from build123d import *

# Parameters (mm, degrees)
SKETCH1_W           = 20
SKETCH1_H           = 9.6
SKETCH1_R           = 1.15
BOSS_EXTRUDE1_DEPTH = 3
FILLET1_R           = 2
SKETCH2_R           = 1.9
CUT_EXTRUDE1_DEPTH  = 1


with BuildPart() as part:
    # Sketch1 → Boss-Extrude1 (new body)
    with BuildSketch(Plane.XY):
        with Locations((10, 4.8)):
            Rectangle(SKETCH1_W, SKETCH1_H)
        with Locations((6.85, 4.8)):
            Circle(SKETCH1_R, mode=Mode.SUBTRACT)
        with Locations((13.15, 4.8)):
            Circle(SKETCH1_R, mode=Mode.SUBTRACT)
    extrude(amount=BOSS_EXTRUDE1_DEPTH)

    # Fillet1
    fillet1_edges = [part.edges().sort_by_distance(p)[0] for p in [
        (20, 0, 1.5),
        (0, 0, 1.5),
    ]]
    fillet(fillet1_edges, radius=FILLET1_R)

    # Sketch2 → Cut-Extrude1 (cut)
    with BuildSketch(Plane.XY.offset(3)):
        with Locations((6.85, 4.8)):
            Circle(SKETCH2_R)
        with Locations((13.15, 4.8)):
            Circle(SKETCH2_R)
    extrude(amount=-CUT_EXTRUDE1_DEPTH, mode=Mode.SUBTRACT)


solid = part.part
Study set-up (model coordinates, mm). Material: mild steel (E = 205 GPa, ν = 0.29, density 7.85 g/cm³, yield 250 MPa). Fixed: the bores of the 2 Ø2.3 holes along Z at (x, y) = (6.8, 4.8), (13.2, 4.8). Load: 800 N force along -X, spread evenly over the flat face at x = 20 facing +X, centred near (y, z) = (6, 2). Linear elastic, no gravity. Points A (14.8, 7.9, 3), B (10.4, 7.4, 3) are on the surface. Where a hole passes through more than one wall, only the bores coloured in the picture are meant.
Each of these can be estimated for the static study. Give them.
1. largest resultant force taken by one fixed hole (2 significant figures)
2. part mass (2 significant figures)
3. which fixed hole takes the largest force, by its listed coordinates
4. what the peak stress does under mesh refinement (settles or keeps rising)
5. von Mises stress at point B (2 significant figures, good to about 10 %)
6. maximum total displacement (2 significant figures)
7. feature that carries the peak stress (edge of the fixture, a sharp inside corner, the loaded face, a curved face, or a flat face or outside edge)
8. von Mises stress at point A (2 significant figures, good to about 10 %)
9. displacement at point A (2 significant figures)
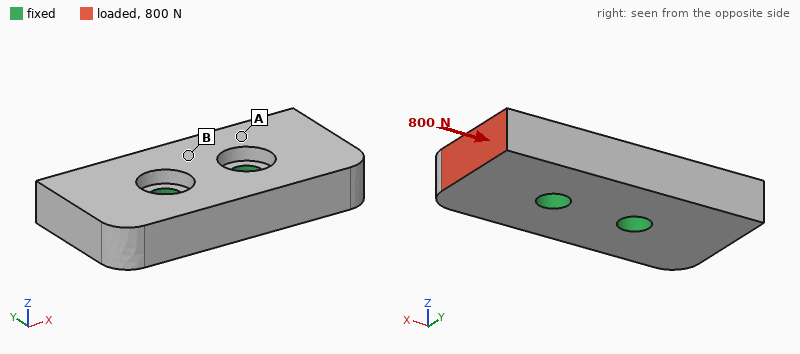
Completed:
620 N
4.2 g
(13.2, 4.8)
keeps rising
21 MPa
3.0 µm
edge of the fixture
43 MPa
1.3 µm
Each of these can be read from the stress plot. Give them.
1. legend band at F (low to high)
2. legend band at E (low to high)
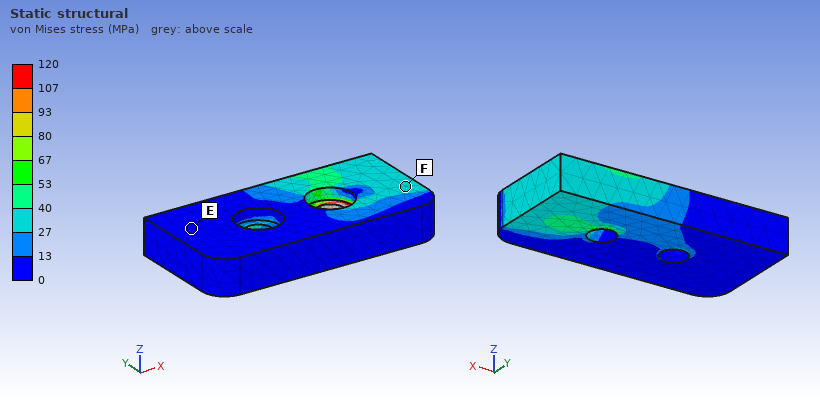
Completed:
27 to 40 MPa
0 to 13 MPa
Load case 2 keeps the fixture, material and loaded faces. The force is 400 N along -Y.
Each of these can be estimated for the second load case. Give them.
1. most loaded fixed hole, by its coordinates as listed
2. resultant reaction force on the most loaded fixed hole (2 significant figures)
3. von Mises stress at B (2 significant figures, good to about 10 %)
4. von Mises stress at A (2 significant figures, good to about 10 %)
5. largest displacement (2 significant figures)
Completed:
(13.2, 4.8)
660 N
16 MPa
29 MPa
5.6 µm
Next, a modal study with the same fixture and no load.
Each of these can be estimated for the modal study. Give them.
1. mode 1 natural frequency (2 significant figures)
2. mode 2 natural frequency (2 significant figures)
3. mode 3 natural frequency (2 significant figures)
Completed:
38 kHz
39 kHz
46 kHz
